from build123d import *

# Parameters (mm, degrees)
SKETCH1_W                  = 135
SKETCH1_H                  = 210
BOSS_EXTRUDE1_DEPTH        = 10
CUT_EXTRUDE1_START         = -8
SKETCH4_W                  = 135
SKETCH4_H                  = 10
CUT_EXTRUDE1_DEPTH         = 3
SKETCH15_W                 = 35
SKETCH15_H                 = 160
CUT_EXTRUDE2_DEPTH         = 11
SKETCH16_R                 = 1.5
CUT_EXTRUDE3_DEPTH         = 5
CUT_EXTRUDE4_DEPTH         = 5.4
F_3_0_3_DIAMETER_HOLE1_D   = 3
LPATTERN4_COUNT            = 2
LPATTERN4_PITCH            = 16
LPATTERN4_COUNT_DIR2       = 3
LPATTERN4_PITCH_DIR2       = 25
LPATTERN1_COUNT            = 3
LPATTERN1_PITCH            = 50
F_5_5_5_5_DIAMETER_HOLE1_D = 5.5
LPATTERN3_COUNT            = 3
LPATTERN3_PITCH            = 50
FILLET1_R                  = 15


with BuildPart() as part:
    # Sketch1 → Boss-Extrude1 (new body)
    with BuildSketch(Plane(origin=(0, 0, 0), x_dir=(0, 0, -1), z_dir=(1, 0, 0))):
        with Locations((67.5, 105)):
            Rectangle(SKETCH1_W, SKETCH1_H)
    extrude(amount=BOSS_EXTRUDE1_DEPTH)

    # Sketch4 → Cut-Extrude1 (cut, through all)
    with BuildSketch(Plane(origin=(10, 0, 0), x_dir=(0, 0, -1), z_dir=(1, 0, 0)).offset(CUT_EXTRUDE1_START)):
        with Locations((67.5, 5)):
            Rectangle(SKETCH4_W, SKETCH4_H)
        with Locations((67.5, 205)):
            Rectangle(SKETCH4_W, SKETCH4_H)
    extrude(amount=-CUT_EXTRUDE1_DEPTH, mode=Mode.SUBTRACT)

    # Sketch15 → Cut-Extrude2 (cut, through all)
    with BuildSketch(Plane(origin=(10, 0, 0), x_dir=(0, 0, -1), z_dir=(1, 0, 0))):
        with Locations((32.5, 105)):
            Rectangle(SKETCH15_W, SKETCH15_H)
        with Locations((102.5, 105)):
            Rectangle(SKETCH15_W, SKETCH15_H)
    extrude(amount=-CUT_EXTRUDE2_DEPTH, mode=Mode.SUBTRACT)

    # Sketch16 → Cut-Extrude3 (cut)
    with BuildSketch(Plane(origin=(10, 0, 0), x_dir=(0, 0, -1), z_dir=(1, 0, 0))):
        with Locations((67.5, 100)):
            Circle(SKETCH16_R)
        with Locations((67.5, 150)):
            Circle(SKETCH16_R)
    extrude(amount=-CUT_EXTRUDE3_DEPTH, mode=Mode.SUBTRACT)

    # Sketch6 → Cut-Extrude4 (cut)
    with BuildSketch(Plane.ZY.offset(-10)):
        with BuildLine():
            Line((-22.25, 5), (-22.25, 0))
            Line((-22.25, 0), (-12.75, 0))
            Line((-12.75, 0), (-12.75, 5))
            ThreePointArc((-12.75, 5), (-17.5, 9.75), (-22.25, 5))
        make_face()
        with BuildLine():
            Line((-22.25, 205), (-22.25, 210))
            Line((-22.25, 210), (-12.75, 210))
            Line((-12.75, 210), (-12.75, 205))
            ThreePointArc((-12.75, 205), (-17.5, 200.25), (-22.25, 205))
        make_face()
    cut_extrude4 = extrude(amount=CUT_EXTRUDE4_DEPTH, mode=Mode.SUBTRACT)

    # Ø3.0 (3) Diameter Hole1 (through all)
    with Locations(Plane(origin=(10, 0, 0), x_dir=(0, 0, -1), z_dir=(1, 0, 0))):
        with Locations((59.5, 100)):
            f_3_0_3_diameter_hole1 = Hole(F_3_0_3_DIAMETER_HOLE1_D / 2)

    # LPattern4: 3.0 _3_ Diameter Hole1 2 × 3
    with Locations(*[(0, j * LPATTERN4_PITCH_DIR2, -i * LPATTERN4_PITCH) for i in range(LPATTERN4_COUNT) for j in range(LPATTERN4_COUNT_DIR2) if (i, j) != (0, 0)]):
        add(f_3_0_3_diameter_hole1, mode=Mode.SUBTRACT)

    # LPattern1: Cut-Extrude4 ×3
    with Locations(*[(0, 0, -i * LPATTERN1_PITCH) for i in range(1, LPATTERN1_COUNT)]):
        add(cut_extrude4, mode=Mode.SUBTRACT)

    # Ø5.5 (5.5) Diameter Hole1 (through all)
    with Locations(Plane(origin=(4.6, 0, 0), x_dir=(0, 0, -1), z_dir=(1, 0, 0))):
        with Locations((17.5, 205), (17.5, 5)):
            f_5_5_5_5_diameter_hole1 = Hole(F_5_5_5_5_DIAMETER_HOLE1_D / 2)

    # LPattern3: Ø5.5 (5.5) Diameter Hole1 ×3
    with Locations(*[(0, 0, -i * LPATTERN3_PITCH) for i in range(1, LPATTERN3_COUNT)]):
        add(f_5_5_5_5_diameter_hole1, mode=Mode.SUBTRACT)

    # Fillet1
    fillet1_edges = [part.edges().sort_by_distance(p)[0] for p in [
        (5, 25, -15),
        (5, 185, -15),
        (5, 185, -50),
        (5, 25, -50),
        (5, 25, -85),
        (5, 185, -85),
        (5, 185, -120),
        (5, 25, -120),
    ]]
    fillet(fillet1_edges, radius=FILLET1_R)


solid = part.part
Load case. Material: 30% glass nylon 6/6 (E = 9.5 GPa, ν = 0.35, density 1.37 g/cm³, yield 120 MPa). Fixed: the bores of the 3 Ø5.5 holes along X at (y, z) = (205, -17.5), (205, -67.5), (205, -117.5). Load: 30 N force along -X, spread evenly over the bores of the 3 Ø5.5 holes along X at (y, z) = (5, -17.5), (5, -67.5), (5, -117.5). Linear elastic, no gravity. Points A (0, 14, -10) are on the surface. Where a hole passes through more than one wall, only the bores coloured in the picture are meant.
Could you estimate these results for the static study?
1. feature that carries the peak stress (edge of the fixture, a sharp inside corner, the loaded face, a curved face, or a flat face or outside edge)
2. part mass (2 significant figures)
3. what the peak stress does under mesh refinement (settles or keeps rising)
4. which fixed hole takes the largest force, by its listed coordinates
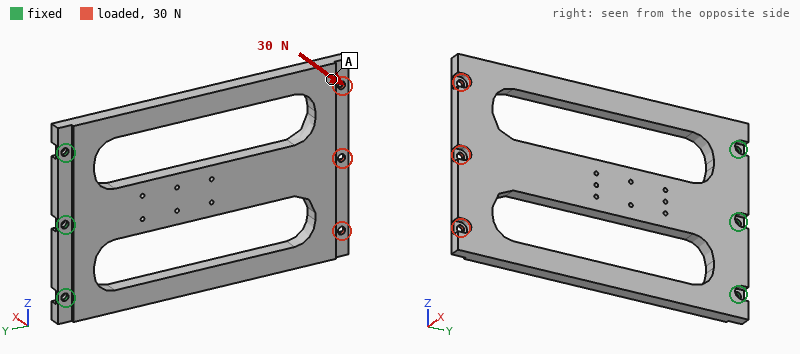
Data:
edge of the fixture
230 g
keeps rising
(205, -67.5)
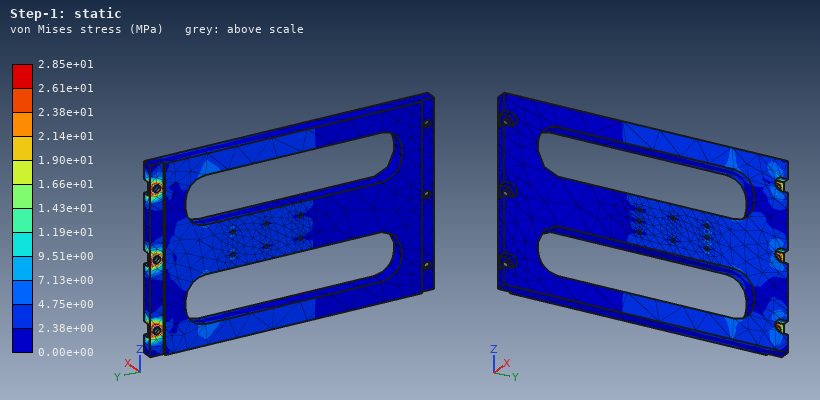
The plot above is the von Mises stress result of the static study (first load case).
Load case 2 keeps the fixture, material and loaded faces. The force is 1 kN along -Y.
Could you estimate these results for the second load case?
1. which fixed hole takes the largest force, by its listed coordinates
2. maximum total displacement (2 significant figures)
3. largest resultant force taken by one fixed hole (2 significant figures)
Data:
(205, -67.5)
0.66 mm
380 N
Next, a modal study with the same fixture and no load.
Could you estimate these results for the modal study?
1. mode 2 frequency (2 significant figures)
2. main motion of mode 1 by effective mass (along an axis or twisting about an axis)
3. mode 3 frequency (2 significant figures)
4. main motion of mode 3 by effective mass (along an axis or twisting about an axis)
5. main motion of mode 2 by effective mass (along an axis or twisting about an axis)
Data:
240 Hz
along X
410 Hz
along Z
twisting about Y
